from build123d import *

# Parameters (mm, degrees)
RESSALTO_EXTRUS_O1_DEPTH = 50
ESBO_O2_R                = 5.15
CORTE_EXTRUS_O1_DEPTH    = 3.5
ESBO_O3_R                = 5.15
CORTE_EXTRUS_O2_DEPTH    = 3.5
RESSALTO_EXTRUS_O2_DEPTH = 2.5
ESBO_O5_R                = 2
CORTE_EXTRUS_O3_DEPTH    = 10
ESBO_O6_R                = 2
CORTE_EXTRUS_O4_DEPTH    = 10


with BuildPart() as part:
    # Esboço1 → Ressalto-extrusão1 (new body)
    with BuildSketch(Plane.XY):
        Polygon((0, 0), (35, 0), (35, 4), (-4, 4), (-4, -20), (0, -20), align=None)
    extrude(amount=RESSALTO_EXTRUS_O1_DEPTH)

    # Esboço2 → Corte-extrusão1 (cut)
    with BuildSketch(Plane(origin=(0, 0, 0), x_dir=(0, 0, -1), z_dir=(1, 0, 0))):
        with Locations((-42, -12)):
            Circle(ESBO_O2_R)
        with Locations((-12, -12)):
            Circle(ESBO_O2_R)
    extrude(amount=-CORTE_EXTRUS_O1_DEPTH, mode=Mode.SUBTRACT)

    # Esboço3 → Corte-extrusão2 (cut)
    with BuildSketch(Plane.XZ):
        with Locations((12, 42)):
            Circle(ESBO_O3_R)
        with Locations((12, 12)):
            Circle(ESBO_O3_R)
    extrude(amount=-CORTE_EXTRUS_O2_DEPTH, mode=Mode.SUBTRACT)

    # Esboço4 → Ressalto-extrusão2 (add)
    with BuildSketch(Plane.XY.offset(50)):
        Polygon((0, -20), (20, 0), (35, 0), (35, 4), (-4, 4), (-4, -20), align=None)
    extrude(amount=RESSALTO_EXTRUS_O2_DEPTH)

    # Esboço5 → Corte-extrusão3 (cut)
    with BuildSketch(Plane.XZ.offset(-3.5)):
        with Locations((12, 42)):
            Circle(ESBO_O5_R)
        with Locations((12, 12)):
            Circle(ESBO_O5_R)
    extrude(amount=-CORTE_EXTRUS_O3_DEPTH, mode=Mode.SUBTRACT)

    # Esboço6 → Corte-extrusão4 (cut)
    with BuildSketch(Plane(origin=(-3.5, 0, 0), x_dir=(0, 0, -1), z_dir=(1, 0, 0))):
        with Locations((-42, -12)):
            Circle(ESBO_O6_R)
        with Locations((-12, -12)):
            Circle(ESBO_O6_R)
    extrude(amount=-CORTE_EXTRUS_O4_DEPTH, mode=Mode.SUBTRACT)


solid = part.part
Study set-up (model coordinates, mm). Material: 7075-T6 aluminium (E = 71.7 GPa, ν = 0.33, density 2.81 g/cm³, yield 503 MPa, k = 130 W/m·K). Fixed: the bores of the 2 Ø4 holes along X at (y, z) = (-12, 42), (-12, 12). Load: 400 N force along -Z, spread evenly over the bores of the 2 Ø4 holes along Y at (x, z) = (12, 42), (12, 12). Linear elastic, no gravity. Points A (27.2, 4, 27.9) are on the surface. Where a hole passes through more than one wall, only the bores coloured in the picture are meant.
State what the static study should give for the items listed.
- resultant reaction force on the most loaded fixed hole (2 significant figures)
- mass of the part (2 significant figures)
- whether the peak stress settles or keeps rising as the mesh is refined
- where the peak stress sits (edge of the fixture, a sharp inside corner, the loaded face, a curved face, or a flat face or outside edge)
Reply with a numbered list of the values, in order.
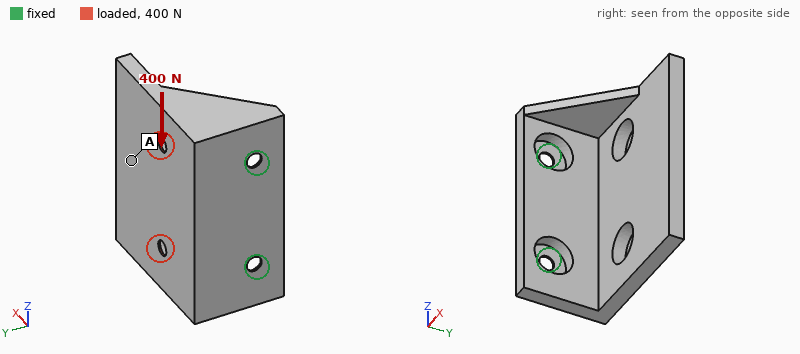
1. 360 N
2. 33 g
3. keeps rising
4. edge of the fixture
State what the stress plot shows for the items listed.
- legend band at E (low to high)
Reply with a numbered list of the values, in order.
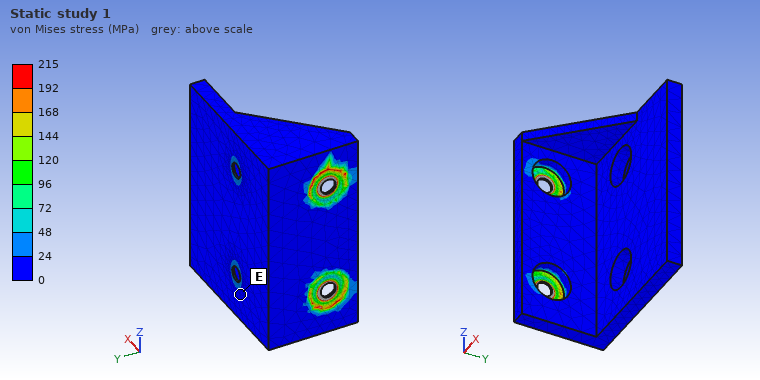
1. 0 to 24 MPa
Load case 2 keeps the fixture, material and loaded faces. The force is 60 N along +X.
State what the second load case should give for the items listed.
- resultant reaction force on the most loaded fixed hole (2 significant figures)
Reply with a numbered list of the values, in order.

1. 31 N
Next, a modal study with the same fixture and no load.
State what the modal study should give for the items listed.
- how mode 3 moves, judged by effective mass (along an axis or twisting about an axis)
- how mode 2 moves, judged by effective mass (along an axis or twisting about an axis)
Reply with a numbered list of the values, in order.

1. along X
2. along Z
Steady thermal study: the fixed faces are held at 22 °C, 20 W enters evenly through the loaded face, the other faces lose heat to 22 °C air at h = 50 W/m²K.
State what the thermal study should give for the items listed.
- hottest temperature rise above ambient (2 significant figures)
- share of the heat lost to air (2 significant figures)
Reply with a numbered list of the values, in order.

1. 54 K
2. 43 %
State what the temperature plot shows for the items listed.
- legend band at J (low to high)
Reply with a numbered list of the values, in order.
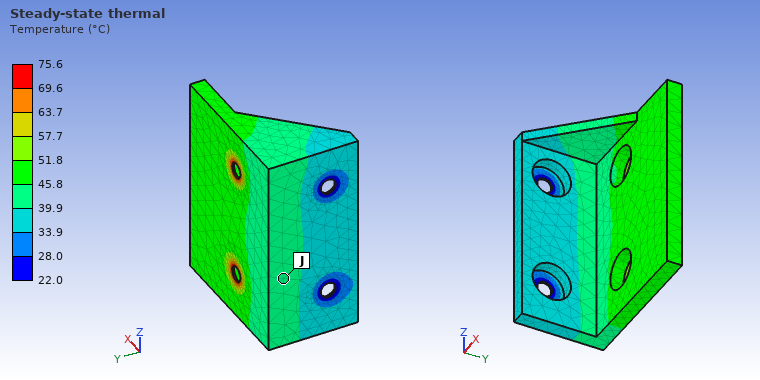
1. 39.9 to 45.8 °C
